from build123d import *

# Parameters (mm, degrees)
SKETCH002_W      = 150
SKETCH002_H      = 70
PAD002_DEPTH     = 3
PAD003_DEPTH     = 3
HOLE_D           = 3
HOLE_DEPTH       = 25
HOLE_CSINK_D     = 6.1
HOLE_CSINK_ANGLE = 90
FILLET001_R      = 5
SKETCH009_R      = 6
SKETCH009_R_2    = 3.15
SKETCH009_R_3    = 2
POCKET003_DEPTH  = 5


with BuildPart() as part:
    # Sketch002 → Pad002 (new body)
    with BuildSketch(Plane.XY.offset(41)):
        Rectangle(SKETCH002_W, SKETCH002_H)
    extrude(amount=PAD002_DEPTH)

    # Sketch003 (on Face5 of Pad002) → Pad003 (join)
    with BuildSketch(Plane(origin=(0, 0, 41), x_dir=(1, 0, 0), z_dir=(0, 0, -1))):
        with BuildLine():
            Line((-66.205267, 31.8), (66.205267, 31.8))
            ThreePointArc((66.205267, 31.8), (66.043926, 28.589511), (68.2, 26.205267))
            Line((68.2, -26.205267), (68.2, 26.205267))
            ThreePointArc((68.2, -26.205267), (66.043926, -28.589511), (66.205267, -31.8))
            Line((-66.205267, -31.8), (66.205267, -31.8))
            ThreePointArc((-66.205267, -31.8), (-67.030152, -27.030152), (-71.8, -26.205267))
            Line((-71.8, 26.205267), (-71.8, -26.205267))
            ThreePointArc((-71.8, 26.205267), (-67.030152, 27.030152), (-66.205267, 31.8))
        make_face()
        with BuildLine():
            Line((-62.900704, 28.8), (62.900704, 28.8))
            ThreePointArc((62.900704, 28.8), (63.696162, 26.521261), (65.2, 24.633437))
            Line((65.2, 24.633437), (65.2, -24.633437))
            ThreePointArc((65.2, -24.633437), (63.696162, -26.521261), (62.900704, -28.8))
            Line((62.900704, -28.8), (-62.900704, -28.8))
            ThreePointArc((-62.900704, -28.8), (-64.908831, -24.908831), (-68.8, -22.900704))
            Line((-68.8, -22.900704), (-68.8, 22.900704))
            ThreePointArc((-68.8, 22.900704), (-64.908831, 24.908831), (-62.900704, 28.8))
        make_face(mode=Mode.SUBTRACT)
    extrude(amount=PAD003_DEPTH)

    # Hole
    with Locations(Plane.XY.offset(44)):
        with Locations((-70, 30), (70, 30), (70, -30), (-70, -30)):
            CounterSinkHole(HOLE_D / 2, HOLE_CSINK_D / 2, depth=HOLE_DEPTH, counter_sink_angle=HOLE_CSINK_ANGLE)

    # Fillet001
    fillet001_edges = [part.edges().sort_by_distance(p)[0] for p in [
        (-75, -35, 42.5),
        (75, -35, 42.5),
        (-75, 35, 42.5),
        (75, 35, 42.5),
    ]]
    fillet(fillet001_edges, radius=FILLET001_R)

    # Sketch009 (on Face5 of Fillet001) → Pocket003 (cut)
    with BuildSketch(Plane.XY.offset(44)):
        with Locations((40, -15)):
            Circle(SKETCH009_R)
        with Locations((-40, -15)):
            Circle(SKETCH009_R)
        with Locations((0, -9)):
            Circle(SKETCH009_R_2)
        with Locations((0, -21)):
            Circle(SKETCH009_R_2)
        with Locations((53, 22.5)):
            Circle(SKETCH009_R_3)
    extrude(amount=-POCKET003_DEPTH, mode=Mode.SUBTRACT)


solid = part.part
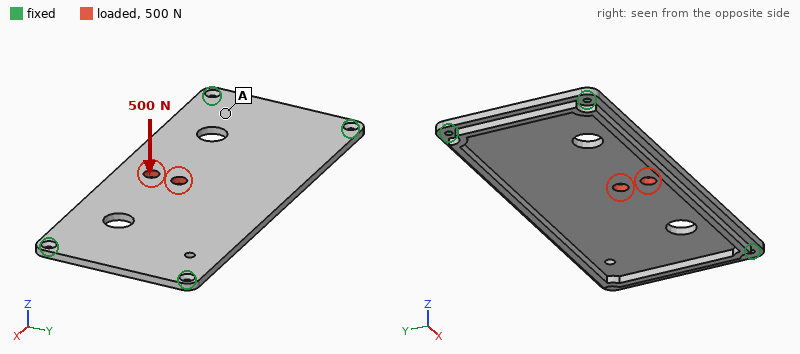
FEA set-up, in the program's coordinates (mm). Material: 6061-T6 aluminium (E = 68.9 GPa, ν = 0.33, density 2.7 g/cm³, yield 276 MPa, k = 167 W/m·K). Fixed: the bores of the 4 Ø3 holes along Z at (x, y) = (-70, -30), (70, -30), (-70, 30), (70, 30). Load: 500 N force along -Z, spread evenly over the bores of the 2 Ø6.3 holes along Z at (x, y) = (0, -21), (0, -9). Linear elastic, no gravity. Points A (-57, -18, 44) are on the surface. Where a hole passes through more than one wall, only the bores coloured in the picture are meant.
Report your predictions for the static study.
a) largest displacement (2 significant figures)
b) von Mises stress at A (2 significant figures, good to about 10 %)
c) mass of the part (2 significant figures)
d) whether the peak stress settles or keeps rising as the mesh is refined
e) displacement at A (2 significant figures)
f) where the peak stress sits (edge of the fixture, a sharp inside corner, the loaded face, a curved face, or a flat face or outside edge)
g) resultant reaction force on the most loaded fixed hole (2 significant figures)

0.83 mm
26 MPa
91 g
keeps rising
0.15 mm
edge of the fixture
230 N
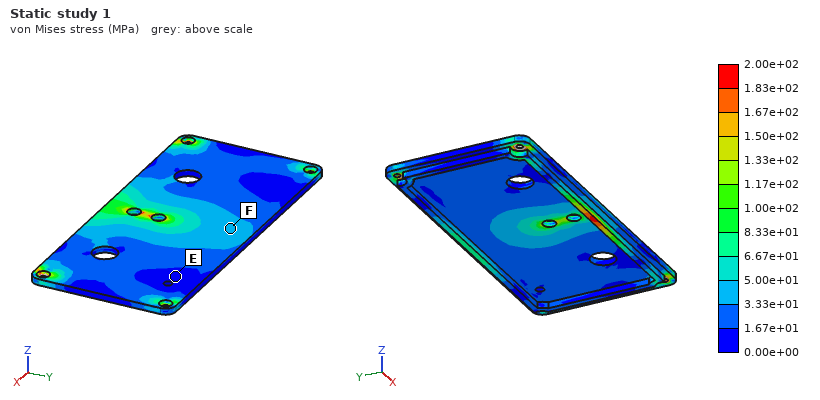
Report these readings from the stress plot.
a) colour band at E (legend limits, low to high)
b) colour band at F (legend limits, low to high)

0.00e+00 to 1.67e+01 MPa
3.33e+01 to 5.00e+01 MPa
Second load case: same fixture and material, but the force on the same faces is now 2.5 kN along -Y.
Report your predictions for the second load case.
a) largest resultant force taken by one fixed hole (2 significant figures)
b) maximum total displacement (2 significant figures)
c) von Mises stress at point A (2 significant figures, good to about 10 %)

940 N
45 µm
14 MPa
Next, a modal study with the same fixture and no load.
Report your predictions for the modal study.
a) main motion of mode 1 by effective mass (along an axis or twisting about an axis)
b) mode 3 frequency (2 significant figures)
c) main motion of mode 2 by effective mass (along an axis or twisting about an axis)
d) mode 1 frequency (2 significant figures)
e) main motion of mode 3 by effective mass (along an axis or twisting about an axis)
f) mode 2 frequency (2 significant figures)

along Z
2200 Hz
twisting about X
730 Hz
twisting about Y
1300 Hz
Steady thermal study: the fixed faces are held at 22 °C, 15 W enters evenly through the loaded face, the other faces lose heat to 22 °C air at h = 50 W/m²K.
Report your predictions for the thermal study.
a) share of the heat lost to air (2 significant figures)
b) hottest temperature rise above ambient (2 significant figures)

48 %
18 K
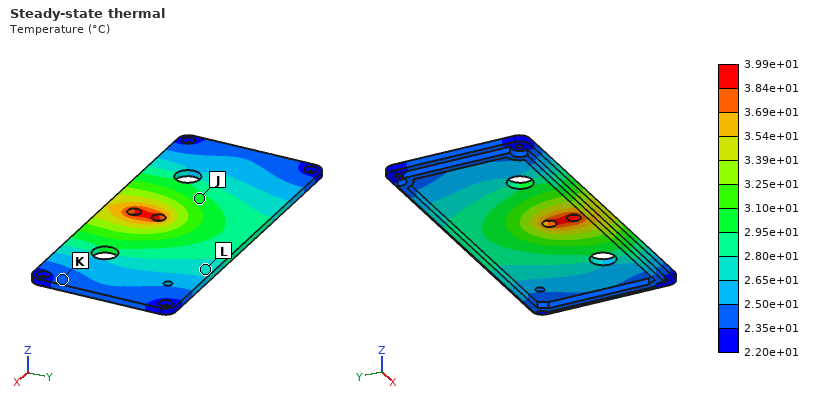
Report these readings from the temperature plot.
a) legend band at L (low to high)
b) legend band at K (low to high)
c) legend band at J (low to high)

2.65e+01 to 2.80e+01 °C
2.35e+01 to 2.50e+01 °C
2.95e+01 to 3.10e+01 °C
